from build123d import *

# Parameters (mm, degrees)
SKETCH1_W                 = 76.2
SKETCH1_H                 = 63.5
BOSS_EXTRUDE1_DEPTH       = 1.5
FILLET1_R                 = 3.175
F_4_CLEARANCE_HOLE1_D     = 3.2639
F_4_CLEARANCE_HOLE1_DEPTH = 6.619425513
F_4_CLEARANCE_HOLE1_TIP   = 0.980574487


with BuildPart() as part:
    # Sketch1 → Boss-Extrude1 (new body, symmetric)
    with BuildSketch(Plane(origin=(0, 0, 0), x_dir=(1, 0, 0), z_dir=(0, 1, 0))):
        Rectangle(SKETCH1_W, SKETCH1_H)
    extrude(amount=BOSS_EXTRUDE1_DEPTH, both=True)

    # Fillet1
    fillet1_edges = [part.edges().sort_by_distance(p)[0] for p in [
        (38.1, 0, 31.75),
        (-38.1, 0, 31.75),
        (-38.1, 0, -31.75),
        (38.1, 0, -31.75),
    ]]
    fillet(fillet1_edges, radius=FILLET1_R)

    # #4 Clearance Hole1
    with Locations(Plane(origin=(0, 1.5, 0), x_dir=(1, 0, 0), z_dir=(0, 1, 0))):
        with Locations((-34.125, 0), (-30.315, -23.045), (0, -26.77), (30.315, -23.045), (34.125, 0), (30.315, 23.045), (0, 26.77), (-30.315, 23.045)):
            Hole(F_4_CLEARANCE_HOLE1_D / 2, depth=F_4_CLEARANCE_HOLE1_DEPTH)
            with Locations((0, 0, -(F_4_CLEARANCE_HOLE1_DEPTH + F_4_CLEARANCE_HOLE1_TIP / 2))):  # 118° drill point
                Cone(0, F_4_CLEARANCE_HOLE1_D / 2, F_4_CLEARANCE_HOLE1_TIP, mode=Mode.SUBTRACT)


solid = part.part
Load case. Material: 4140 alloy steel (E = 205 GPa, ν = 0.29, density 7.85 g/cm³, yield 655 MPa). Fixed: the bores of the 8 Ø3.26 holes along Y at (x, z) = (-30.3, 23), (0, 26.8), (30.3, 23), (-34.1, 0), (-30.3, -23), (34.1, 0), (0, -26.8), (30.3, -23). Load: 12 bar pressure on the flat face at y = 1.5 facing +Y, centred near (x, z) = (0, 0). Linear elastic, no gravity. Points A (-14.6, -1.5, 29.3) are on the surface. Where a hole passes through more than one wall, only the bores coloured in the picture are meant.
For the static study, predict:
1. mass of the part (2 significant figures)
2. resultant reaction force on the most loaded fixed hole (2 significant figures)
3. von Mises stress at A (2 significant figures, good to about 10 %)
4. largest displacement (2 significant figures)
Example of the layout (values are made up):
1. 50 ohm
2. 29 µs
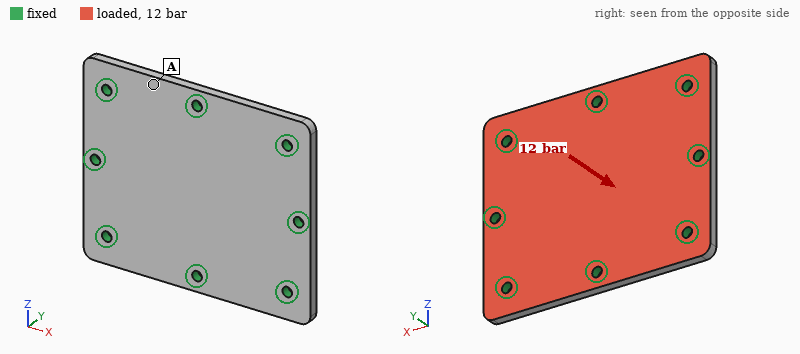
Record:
1. 110 g
2. 1.0 kN
3. 33 MPa
4. 47 µm
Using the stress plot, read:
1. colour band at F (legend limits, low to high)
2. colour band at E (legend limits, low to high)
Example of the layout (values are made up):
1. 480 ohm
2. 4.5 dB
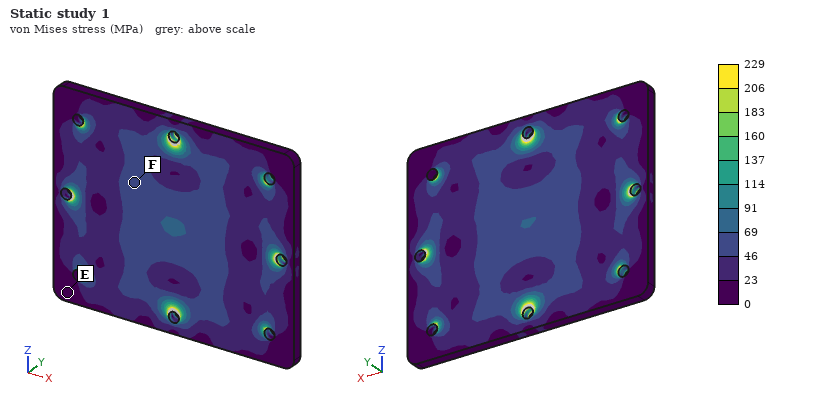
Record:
1. 46 to 69 MPa
2. 0 to 23 MPa
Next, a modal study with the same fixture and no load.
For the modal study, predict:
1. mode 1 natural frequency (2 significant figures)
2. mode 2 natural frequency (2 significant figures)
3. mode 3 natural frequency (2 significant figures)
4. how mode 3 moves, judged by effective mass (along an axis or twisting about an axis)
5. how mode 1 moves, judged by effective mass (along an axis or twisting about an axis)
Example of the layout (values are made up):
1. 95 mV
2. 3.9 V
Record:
1. 6500 Hz
2. 11 kHz
3. 14 kHz
4. twisting about X
5. along Y
